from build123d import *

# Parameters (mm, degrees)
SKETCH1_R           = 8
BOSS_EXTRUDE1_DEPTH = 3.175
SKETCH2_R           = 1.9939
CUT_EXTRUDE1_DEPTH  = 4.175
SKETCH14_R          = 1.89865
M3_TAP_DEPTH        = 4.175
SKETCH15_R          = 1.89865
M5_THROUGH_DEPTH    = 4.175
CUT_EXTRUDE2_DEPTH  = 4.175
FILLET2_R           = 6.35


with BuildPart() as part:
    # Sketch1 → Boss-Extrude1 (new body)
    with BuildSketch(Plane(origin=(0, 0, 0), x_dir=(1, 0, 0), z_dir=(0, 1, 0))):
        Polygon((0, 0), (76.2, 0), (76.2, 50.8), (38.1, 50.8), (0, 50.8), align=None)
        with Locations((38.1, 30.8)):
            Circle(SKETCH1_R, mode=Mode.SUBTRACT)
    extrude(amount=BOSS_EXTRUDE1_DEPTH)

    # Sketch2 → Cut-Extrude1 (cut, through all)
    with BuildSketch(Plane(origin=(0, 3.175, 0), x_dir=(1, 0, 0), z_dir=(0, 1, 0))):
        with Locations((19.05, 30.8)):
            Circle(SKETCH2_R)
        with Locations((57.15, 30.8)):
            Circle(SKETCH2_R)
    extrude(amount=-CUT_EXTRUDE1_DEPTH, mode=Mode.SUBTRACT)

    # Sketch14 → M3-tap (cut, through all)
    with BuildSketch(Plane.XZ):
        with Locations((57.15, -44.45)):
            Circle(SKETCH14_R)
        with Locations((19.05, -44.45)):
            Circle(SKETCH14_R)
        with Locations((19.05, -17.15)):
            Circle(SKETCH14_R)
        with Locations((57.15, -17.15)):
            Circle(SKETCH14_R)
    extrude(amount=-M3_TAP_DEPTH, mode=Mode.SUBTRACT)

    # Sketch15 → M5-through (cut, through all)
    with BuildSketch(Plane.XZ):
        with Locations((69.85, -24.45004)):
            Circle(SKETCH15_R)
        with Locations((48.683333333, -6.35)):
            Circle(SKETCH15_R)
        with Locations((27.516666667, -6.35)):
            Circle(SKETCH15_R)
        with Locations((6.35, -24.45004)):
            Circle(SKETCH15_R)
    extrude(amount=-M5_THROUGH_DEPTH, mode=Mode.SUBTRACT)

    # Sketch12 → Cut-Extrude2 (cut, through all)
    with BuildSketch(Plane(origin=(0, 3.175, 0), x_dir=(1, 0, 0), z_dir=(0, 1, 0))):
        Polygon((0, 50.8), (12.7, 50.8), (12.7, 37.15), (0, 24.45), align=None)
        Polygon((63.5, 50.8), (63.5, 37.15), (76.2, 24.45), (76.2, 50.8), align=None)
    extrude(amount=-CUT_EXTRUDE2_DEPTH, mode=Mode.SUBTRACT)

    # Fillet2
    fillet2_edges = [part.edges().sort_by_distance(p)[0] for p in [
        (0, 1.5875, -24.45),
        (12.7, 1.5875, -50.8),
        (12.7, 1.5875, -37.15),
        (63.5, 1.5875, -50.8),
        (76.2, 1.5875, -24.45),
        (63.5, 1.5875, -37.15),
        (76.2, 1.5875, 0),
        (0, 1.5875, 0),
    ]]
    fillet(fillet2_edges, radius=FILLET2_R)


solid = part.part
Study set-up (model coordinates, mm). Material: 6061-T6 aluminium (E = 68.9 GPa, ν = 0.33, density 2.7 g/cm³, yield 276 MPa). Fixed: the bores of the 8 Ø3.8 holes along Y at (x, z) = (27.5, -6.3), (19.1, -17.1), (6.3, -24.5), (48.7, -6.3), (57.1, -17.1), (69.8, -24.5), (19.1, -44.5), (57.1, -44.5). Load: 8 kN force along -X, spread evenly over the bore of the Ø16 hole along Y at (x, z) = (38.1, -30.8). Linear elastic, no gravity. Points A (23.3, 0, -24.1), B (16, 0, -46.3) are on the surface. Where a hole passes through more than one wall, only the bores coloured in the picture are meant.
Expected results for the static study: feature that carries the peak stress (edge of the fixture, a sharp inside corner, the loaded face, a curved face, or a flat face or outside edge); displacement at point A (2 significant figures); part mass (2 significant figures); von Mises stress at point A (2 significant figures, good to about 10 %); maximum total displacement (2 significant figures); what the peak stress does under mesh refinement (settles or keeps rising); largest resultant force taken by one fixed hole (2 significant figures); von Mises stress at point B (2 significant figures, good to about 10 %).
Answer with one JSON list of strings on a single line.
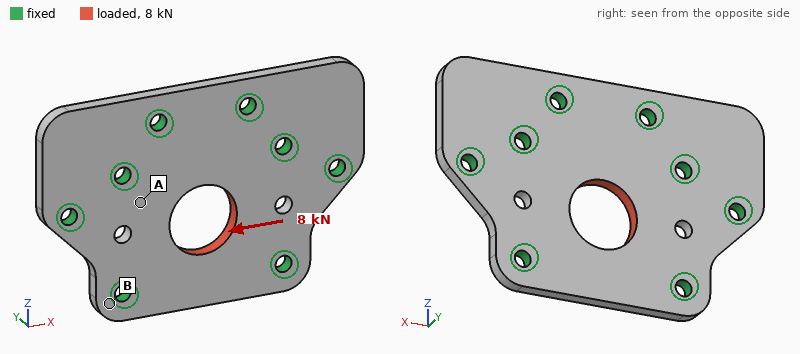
["edge of the fixture", "5.7 µm", "26 g", "40 MPa", "13 µm", "keeps rising", "1.8 kN", "18 MPa"]
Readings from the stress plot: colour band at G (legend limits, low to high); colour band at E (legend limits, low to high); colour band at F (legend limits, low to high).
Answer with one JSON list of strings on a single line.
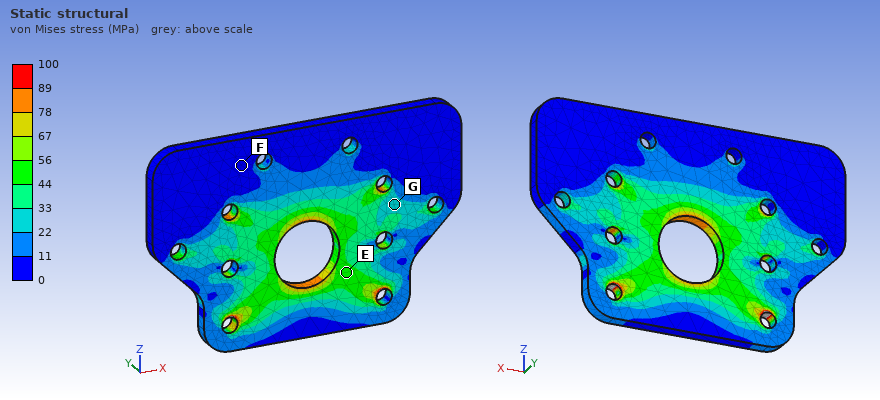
["22 to 33 MPa", "44 to 56 MPa", "0 to 11 MPa"]
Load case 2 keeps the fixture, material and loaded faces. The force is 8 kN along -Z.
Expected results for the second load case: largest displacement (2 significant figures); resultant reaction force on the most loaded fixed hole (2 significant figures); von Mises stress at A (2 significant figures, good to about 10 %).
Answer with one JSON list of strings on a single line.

["27 µm", "1.5 kN", "46 MPa"]
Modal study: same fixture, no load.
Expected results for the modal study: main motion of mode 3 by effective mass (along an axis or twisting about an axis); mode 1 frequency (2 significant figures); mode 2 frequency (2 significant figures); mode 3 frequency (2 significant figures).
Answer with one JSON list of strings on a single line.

["along Y", "9000 Hz", "9000 Hz", "12 kHz"]
